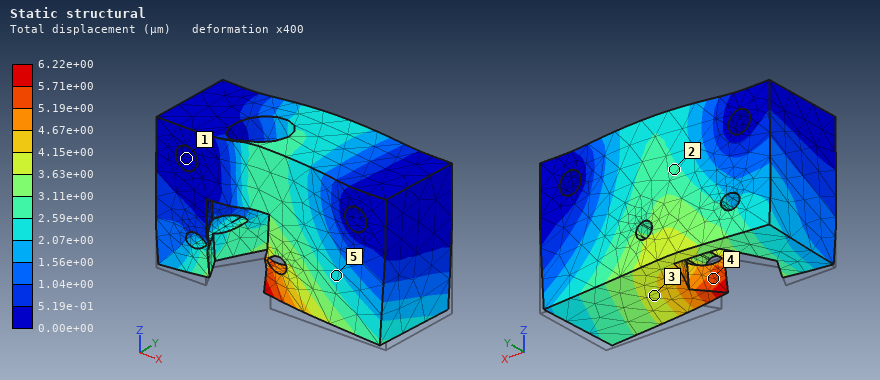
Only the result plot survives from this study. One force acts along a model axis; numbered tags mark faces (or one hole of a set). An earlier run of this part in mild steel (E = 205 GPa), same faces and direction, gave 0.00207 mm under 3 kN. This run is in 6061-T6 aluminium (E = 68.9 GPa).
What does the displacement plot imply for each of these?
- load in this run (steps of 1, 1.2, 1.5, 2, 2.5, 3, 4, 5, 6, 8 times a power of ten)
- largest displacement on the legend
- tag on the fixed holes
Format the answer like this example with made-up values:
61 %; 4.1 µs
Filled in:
3 kN; 6.22e+00 µm; 1
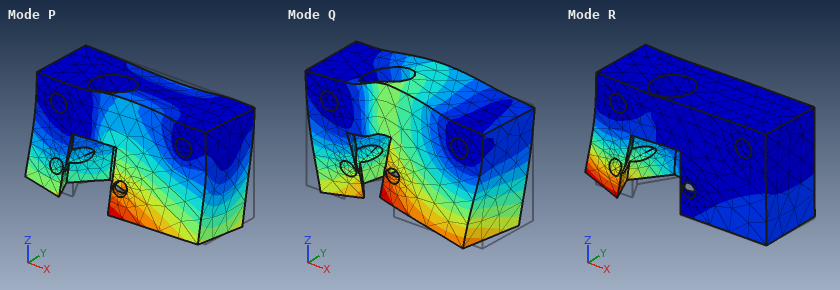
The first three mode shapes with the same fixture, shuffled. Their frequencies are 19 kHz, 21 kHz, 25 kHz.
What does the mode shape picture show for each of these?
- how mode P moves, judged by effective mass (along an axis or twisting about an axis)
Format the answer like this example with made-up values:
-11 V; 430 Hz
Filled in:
along Y
